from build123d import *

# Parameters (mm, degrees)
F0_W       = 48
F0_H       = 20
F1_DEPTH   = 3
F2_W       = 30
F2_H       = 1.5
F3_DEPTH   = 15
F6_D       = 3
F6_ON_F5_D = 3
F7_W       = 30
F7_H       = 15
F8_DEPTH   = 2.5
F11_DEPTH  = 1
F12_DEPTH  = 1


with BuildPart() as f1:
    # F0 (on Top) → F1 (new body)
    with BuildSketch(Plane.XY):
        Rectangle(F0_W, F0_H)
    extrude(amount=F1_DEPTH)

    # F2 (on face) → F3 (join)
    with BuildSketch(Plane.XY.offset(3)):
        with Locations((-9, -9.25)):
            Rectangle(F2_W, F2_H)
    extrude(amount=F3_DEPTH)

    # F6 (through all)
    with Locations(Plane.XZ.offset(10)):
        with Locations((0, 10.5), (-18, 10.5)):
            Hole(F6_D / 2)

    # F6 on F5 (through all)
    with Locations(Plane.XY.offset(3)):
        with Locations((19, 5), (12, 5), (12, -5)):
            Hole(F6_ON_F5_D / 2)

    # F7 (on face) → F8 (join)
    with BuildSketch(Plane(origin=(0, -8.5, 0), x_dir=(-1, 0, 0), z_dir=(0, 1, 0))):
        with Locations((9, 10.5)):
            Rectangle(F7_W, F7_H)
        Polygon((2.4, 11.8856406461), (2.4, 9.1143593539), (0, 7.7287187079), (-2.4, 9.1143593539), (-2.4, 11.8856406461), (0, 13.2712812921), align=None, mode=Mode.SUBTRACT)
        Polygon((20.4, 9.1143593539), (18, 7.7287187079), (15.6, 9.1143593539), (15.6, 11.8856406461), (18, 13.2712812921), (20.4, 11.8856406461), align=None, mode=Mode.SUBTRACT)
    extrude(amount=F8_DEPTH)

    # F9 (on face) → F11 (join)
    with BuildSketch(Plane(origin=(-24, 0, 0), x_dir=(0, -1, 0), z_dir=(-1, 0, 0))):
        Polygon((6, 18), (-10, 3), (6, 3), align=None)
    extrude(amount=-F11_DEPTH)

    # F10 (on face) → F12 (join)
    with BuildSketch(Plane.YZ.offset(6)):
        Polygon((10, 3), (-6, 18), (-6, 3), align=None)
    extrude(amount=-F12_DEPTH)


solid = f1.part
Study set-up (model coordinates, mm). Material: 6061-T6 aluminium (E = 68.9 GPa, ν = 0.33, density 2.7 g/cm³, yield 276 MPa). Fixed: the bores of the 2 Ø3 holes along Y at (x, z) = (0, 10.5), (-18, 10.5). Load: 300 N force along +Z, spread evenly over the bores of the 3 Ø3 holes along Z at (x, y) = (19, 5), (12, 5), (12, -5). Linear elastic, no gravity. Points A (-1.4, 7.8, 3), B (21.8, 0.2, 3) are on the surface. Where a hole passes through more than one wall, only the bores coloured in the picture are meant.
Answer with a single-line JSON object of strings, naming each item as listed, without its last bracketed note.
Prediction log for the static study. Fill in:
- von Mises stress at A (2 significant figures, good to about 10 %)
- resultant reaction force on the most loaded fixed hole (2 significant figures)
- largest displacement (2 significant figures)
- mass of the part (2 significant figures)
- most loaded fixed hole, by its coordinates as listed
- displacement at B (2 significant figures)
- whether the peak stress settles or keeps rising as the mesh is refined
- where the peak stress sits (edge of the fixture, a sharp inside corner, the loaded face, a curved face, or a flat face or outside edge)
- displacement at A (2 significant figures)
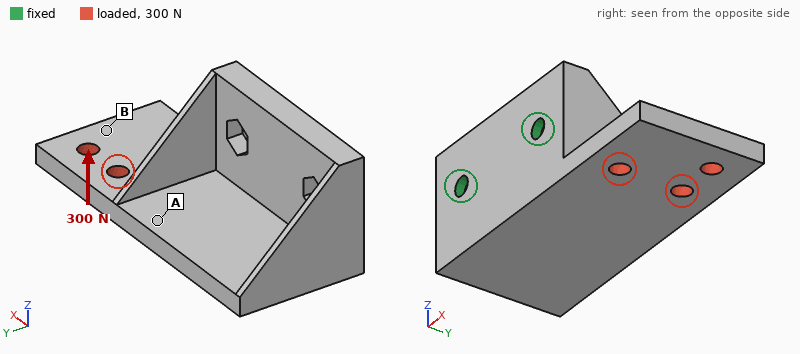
{"von Mises stress at A": "43 MPa", "resultant reaction force on the most loaded fixed hole": "510 N", "largest displacement": "0.33 mm", "mass of the part": "13 g", "most loaded fixed hole, by its coordinates as listed": "(0, 10.5)", "displacement at B": "0.21 mm", "whether the peak stress settles or keeps rising as the mesh is refined": "keeps rising", "where the peak stress sits": "edge of the fixture", "displacement at A": "0.088 mm"}
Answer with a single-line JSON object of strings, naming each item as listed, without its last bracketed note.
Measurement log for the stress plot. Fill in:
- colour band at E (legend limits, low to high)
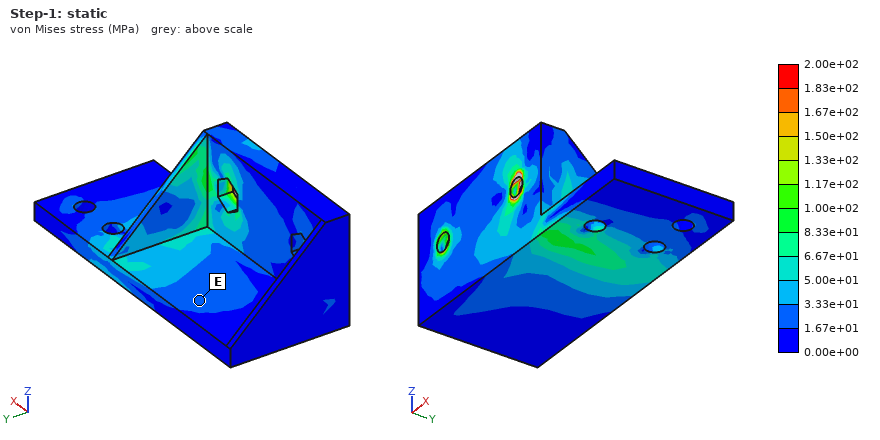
{"colour band at E": "1.67e+01 to 3.33e+01 MPa"}
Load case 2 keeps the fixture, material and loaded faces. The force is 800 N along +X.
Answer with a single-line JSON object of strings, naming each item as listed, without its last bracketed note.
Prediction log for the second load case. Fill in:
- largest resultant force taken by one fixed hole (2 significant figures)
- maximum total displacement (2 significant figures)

{"largest resultant force taken by one fixed hole": "720 N", "maximum total displacement": "0.10 mm"}
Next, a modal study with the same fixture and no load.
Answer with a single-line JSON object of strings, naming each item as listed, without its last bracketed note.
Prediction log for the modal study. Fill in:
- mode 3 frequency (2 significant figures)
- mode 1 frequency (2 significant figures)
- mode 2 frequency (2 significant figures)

{"mode 3 frequency": "6300 Hz", "mode 1 frequency": "3200 Hz", "mode 2 frequency": "5000 Hz"}
